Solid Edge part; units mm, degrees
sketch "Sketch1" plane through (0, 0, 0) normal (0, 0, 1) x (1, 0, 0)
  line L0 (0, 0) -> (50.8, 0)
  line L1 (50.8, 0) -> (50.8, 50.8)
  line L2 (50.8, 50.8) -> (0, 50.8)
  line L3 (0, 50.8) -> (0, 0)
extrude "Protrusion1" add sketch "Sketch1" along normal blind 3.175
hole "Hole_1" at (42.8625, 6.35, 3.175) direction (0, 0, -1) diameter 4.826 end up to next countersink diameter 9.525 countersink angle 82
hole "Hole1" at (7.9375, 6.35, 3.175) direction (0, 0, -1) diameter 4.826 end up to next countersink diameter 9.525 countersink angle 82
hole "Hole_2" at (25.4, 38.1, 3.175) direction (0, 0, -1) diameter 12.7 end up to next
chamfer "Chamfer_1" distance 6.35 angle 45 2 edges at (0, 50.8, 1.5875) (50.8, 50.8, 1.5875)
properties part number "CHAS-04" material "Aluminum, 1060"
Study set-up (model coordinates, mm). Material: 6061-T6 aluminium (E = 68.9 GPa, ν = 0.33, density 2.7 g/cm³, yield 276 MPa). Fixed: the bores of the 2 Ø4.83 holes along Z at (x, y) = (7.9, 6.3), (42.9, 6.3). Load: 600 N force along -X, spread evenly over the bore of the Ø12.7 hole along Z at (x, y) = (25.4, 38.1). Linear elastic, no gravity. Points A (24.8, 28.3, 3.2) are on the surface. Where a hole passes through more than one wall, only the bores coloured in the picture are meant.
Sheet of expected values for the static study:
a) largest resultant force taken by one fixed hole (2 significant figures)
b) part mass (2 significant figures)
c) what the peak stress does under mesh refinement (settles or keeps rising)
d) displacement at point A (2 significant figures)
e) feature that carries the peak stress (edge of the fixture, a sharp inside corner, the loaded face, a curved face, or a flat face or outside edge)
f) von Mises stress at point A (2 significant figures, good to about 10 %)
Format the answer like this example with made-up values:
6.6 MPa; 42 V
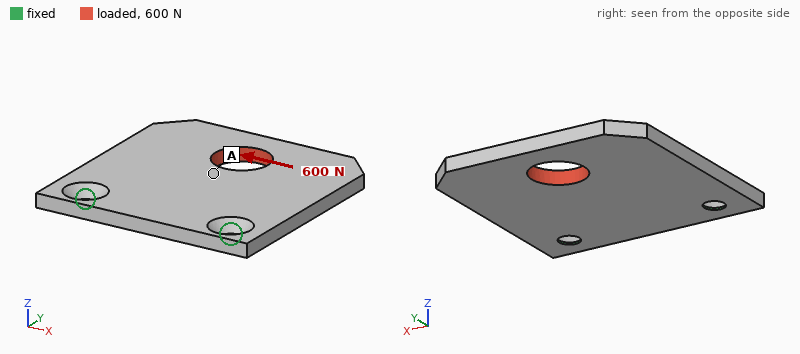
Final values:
590 N; 20 g; keeps rising; 9.0 µm; edge of the fixture; 13 MPa
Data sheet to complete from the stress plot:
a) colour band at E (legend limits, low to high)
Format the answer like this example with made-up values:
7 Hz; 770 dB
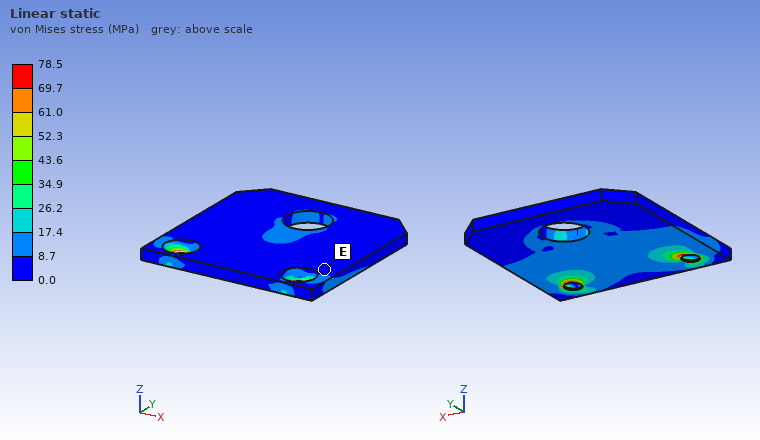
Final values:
0.0 to 8.7 MPa
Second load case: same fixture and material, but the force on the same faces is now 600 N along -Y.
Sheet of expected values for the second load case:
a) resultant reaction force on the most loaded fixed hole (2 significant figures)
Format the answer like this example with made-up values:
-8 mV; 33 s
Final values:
300 N
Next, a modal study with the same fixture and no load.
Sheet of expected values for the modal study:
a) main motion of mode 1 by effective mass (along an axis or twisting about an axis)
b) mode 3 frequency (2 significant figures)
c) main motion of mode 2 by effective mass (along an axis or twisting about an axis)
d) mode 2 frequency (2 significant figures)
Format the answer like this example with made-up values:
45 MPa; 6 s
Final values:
along Z; 6200 Hz; twisting about Y; 2600 Hz
